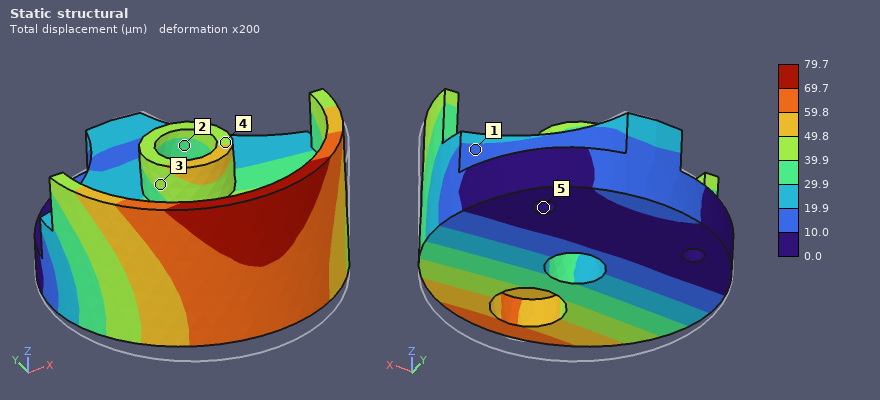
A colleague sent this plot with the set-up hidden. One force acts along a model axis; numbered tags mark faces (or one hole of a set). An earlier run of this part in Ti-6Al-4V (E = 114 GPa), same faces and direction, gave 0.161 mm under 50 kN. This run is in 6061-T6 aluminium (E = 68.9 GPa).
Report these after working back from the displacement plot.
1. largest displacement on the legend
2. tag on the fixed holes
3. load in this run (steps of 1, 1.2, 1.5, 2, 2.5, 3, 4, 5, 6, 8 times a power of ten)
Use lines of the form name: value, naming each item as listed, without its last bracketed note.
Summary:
largest displacement on the legend: 79.7 µm
tag on the fixed holes: 5
load in this run: 15 kN
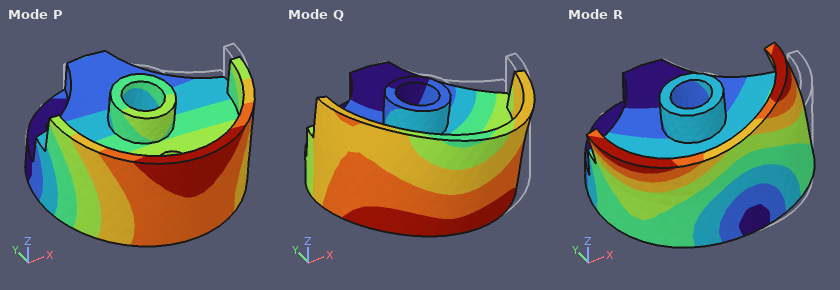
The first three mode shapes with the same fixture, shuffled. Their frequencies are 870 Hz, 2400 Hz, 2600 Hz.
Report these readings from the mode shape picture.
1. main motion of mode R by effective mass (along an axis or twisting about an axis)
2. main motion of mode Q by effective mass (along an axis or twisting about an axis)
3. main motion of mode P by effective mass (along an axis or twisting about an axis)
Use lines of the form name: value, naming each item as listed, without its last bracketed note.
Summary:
main motion of mode R by effective mass: along X
main motion of mode Q by effective mass: along X
main motion of mode P by effective mass: along Z
